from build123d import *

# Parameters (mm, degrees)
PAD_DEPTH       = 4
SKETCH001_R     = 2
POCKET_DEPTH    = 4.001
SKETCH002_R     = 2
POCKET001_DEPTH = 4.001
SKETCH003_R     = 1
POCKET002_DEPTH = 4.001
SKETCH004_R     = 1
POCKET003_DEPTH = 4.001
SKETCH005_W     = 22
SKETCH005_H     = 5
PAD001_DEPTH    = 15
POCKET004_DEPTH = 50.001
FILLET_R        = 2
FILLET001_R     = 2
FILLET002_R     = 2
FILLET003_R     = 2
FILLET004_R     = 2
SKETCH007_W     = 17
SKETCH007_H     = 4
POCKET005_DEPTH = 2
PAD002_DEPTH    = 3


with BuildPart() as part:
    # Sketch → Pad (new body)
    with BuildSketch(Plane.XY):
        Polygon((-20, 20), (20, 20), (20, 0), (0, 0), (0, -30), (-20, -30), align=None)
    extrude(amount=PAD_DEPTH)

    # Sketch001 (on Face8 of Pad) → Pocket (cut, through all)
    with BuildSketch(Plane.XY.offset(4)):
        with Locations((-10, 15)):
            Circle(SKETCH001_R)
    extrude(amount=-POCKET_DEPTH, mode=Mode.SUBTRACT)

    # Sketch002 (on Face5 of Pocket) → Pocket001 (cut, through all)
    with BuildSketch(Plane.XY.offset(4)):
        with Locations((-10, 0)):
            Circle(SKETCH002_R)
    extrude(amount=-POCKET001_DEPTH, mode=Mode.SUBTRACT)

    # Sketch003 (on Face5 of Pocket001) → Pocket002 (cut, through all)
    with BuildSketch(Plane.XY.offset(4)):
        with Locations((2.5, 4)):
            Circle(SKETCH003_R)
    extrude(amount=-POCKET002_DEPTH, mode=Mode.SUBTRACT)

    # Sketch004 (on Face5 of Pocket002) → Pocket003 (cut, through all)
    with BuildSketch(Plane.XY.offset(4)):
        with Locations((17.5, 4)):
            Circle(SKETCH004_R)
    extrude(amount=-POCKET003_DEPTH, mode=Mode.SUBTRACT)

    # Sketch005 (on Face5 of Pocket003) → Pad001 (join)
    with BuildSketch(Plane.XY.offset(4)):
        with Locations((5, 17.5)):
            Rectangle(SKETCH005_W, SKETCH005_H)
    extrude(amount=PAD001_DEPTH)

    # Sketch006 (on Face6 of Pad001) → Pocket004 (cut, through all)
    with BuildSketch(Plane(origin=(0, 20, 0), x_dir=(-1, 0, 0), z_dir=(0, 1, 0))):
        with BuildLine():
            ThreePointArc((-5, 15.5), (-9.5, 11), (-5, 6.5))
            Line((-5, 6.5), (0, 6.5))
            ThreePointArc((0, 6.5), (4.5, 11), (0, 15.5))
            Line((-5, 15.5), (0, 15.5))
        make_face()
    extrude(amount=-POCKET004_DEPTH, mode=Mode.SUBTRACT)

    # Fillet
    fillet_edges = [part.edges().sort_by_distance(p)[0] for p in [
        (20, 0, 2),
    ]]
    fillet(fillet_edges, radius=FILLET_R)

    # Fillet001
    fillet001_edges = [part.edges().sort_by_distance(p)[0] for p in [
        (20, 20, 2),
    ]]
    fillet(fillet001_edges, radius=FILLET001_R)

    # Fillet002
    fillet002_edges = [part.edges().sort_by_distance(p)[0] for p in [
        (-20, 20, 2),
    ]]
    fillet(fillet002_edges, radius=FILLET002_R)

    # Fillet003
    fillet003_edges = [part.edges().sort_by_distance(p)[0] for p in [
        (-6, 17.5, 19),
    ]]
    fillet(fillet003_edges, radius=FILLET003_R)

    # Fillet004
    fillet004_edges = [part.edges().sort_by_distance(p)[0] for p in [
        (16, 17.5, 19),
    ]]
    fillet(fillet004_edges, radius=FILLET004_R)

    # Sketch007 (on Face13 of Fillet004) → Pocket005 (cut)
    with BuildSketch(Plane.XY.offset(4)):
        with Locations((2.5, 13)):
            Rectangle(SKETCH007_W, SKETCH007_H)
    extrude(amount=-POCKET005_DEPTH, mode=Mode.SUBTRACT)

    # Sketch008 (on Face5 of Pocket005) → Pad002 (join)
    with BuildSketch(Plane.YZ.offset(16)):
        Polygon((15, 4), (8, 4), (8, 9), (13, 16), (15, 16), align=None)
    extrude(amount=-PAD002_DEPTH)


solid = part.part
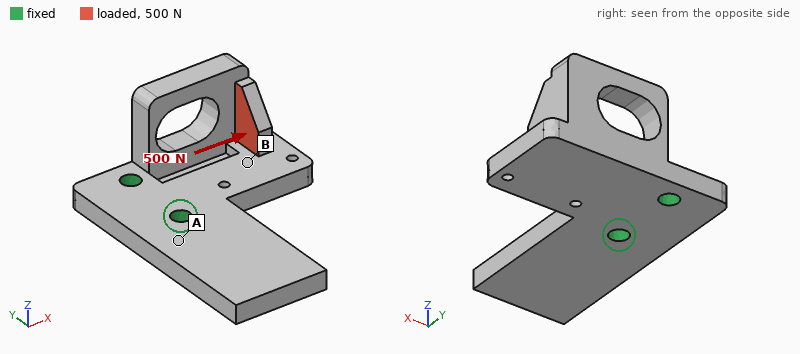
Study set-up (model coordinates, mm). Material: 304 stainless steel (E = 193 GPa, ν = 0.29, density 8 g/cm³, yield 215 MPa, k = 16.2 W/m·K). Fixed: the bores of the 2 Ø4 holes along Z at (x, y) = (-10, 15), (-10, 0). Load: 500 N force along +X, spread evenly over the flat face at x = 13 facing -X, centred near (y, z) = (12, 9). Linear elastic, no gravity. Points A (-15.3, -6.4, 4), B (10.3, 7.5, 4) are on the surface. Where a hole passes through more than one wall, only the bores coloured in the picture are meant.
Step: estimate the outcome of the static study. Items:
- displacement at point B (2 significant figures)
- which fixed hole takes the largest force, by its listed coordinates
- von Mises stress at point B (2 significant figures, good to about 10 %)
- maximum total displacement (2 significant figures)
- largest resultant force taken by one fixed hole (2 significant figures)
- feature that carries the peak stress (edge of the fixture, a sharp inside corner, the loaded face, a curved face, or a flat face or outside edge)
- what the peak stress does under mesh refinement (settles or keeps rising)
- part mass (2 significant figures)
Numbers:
21 µm
(-10, 15)
31 MPa
49 µm
370 N
a sharp inside corner
keeps rising
53 g
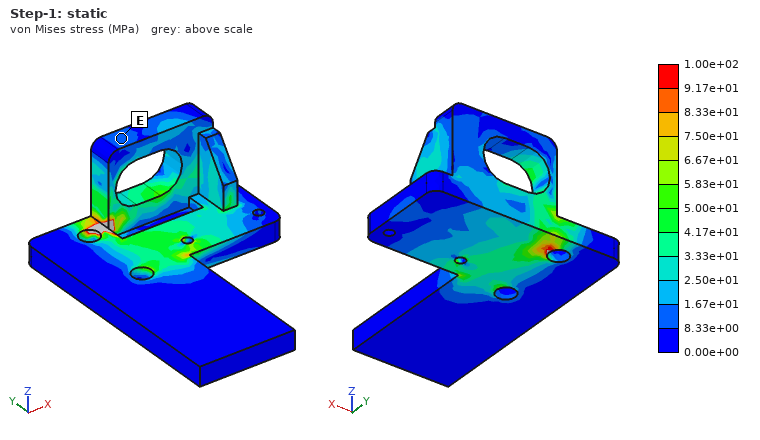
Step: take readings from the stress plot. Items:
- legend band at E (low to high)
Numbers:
8.33e+00 to 1.67e+01 MPa
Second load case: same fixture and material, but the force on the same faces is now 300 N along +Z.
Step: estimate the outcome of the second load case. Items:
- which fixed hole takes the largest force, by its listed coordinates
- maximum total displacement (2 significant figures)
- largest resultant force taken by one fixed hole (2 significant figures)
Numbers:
(-10, 15)
64 µm
210 N
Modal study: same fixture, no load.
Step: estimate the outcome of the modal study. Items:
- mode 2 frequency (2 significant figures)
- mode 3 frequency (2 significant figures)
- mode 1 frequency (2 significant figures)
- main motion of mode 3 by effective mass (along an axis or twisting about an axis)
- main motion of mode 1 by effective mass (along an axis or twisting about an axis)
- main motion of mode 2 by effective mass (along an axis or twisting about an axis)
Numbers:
3600 Hz
5700 Hz
2900 Hz
along Y
along Z
along Z
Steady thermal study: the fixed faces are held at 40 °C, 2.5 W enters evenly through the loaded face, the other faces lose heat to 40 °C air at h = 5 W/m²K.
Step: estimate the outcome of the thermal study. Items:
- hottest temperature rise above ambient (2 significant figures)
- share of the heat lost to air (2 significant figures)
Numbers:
53 K
13 %
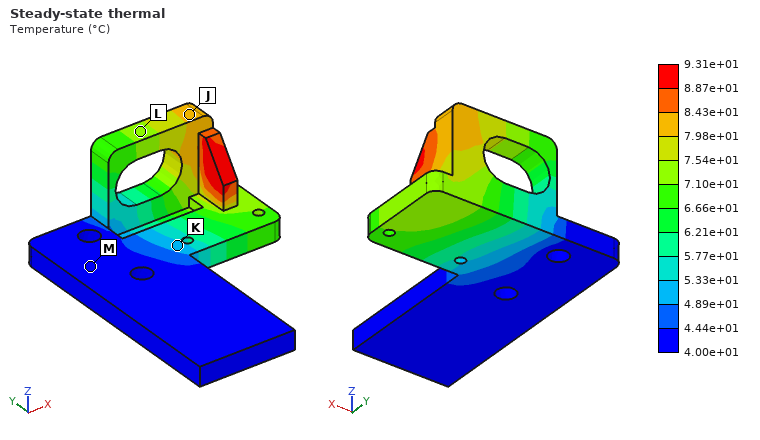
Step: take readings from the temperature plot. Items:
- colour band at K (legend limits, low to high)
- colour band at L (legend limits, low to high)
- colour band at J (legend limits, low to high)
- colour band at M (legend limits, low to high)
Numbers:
4.89e+01 to 5.33e+01 °C
7.10e+01 to 7.54e+01 °C
7.98e+01 to 8.43e+01 °C
4.00e+01 to 4.44e+01 °C
